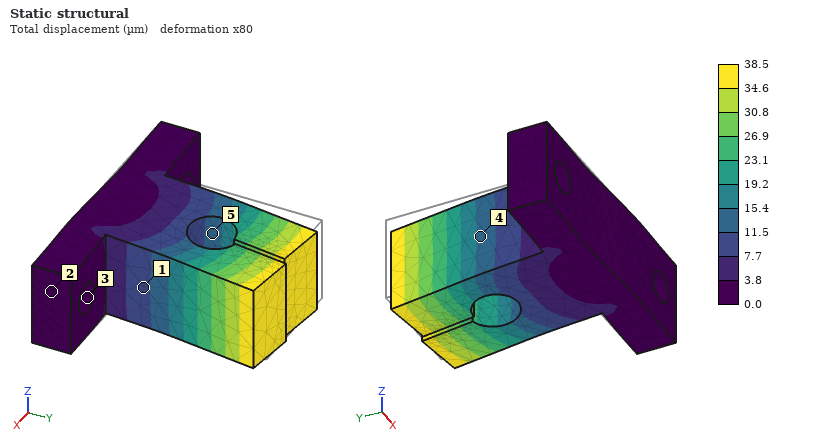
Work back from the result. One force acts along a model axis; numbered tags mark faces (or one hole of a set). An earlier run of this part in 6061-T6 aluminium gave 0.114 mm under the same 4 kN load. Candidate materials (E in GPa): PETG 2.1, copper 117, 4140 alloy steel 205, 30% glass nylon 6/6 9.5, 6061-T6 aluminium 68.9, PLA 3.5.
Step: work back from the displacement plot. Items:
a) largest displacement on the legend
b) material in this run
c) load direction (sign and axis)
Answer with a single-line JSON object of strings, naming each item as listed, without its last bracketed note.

{"largest displacement on the legend": "38.5 µm", "material in this run": "4140 alloy steel", "load direction": "+X"}
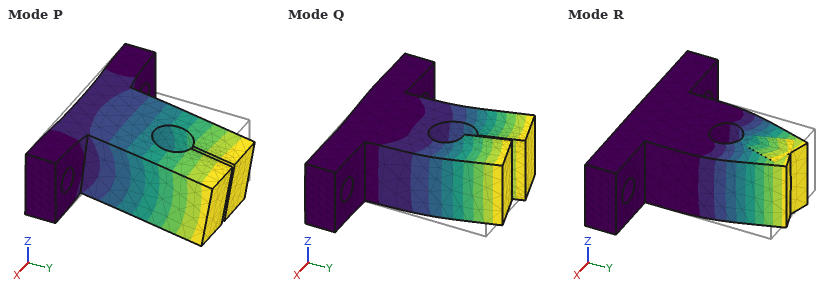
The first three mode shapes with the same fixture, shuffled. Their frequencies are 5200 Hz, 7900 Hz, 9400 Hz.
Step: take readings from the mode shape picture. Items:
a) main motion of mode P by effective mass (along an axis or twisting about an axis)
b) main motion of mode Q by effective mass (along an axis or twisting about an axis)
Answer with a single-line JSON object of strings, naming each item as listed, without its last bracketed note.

{"main motion of mode P by effective mass": "along Z", "main motion of mode Q by effective mass": "along X"}
